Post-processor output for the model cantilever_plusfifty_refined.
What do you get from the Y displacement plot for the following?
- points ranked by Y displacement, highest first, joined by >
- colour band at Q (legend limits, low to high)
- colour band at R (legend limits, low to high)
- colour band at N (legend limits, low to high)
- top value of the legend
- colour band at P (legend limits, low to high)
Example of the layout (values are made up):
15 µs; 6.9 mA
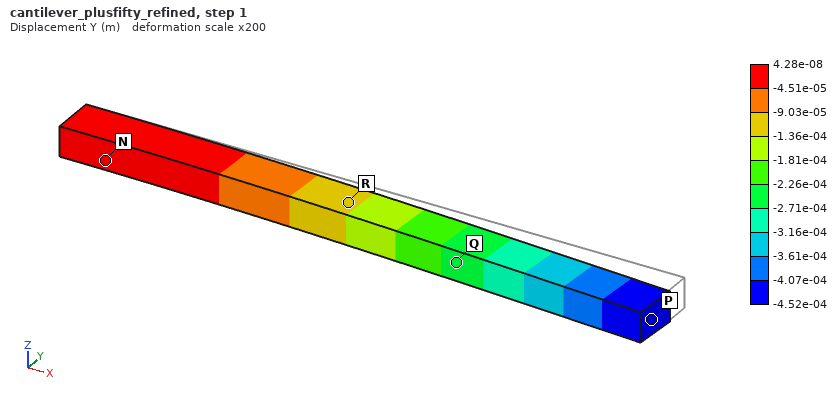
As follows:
N > R > Q > P; -2.71e-04 to -2.26e-04 m; -1.36e-04 to -9.03e-05 m; -4.51e-05 to 4.28e-08 m; 4.28e-08 m; -4.52e-04 to -4.07e-04 m
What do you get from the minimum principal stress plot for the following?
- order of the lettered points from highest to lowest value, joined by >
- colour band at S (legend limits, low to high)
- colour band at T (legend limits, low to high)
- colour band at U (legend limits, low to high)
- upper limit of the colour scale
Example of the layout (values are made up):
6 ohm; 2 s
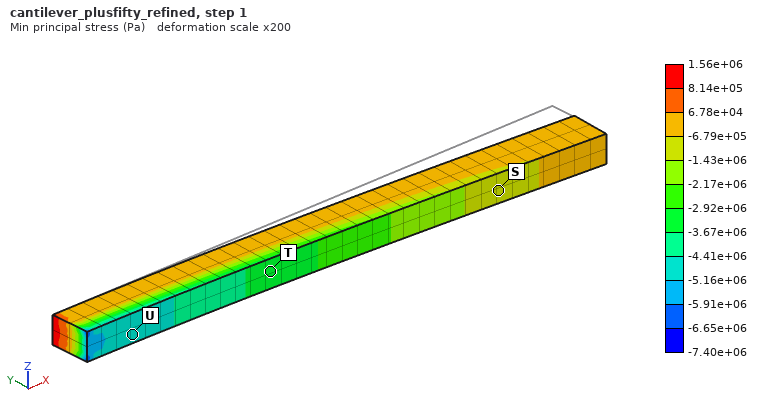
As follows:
S > T > U; -1.43e+06 to -6.79e+05 Pa; -3.67e+06 to -2.92e+06 Pa; -5.16e+06 to -4.41e+06 Pa; 1.56e+06 Pa
